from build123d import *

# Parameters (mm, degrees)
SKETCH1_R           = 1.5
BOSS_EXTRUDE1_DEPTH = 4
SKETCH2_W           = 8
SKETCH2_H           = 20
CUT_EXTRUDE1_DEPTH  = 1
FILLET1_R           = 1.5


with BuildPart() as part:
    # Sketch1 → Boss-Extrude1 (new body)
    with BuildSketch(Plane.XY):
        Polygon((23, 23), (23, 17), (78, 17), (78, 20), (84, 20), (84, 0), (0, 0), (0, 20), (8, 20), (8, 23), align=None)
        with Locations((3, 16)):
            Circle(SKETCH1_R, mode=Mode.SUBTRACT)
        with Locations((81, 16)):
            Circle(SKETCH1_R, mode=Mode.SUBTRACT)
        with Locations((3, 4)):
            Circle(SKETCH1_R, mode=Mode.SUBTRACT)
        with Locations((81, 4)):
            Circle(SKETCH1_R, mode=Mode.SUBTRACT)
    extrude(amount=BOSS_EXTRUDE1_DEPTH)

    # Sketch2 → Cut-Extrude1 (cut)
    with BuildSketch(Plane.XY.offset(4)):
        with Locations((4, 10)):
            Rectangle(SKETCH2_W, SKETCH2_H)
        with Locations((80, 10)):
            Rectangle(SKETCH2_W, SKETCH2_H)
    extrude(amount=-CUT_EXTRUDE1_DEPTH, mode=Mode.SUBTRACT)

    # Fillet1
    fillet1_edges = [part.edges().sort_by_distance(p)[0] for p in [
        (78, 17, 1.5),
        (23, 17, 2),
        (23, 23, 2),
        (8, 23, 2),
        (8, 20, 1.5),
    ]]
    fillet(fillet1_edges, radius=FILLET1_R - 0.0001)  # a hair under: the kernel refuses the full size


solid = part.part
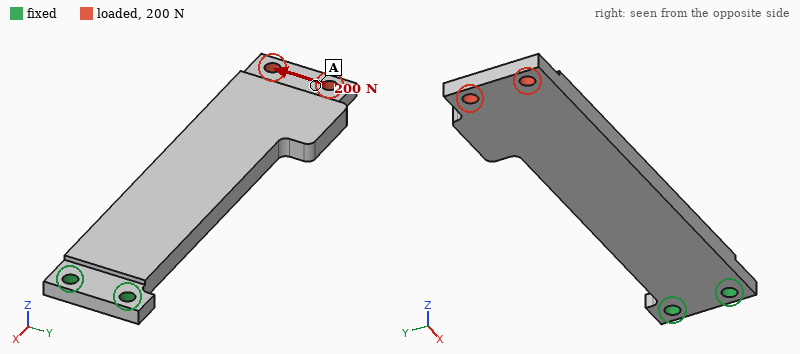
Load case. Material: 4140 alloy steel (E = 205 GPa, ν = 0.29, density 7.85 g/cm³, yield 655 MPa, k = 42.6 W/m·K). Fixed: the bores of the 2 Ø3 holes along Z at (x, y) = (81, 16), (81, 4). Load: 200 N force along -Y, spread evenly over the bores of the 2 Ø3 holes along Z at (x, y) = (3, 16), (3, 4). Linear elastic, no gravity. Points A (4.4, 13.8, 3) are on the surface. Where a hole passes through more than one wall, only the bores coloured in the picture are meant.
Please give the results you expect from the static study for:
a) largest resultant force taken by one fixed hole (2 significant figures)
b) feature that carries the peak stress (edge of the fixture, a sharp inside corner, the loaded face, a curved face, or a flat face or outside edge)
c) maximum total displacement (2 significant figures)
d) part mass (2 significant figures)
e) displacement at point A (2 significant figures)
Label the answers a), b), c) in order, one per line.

a) 1.2 kN
b) a curved face
c) 0.11 mm
d) 46 g
e) 0.100 mm
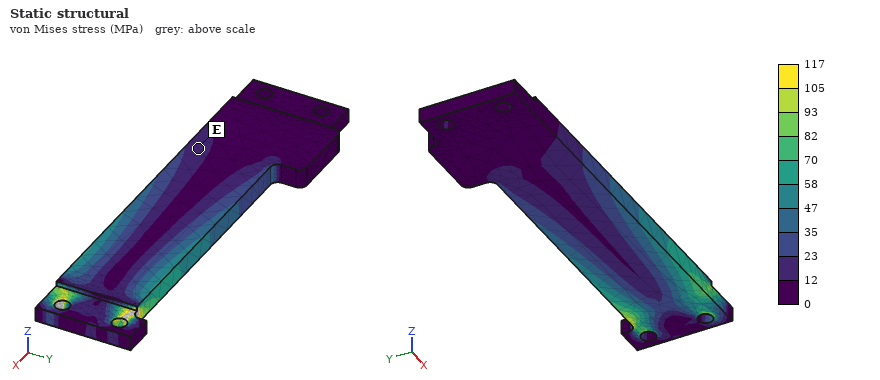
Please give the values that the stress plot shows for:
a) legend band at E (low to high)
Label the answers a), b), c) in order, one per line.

a) 12 to 23 MPa
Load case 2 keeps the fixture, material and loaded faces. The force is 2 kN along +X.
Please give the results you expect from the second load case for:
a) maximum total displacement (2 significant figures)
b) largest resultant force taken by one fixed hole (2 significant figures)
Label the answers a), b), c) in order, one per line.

a) 0.15 mm
b) 1.0 kN
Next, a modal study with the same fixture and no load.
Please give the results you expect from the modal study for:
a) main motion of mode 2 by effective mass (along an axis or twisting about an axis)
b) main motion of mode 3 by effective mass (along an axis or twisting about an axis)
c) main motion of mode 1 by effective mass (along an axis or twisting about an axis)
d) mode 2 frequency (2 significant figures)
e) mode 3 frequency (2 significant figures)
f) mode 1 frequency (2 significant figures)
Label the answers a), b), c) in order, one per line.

a) along Y
b) along Z
c) along Z
d) 1900 Hz
e) 2900 Hz
f) 430 Hz
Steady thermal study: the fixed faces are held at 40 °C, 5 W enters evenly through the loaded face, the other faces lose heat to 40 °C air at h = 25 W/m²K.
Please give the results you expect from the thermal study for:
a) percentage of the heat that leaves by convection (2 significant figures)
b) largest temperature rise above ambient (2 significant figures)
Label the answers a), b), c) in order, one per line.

a) 63 %
b) 76 K
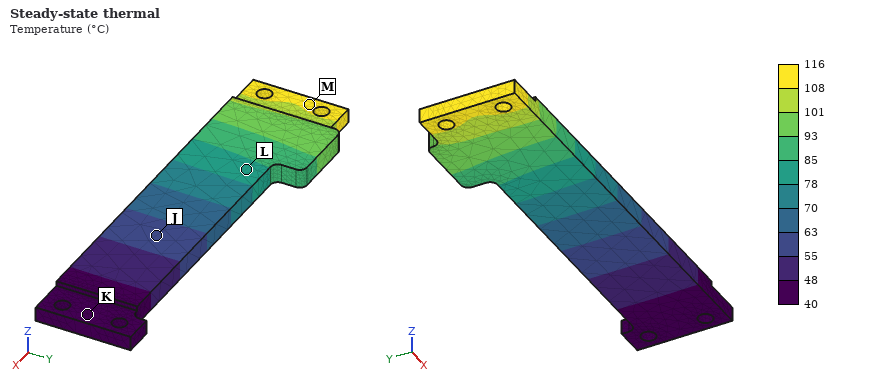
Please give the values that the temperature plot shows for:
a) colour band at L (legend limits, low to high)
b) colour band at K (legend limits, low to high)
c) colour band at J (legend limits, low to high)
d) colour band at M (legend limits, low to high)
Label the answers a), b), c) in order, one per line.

a) 78 to 85 °C
b) 40 to 48 °C
c) 55 to 63 °C
d) 108 to 116 °C
